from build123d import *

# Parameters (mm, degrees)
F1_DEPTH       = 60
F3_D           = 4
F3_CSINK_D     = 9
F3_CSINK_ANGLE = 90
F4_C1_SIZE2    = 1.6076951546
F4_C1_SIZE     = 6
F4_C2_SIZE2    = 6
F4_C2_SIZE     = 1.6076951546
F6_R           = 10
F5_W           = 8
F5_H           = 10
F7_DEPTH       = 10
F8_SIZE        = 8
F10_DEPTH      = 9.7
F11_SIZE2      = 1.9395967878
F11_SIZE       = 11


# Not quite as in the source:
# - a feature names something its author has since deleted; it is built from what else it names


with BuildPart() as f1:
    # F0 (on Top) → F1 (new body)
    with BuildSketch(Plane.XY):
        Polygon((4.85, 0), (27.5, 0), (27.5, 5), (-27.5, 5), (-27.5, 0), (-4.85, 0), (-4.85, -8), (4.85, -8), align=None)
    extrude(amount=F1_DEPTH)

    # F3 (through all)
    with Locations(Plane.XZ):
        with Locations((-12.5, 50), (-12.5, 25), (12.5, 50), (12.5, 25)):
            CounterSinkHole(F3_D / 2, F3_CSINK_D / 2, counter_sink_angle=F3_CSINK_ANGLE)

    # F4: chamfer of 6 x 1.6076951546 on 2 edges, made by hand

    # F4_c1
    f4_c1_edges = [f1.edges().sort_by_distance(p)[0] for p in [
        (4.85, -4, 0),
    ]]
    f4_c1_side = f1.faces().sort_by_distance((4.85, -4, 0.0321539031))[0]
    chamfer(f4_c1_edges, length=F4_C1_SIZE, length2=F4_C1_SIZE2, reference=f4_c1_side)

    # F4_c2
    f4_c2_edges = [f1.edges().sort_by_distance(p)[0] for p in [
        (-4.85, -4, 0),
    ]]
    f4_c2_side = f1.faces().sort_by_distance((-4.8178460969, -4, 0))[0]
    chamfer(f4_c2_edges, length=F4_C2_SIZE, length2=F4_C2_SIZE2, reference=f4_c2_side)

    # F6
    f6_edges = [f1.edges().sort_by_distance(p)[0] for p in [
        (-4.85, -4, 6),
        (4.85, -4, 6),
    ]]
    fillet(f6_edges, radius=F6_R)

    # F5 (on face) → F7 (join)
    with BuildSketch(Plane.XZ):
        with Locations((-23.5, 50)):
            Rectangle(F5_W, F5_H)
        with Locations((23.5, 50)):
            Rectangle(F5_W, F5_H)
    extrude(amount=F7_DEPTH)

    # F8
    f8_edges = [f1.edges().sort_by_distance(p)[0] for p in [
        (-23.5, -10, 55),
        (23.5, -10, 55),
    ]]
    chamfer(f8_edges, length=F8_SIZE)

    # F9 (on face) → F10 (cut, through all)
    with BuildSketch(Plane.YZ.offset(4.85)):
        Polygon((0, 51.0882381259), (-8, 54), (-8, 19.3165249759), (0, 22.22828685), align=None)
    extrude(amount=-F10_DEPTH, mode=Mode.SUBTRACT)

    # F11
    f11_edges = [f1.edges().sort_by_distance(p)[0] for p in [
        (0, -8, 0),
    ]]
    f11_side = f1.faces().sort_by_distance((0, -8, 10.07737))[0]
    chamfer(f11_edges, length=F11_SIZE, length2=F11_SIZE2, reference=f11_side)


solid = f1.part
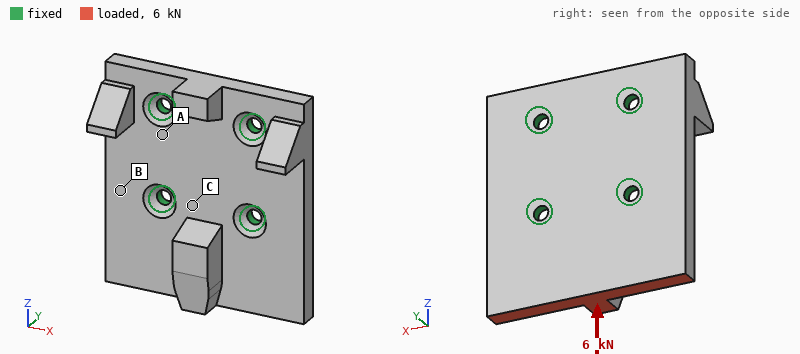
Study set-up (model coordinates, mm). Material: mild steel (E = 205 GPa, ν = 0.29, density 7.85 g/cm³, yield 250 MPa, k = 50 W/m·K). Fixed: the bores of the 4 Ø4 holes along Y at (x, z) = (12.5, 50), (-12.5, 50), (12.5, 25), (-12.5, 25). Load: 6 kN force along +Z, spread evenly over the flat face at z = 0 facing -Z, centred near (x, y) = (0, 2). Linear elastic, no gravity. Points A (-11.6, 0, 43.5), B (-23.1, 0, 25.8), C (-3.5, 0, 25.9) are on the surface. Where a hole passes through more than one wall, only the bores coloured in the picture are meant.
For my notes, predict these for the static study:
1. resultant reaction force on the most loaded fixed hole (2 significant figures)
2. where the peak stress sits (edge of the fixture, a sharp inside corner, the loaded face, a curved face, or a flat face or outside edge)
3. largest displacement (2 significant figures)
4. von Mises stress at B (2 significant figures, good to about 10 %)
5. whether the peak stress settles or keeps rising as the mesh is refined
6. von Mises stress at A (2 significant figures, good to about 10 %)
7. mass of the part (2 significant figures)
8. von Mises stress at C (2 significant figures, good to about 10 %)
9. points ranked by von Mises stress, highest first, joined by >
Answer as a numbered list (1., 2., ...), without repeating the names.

1. 2.1 kN
2. edge of the fixture
3. 19 µm
4. 31 MPa
5. keeps rising
6. 9.1 MPa
7. 150 g
8. 43 MPa
9. C > B > A
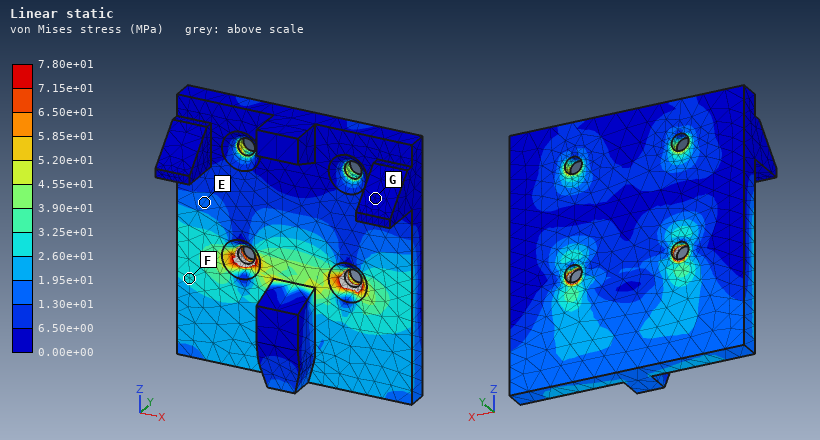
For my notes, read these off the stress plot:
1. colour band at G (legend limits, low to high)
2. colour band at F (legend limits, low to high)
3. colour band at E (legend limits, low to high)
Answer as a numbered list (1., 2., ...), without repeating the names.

1. 0.00e+00 to 6.50e+00 MPa
2. 2.60e+01 to 3.25e+01 MPa
3. 1.30e+01 to 1.95e+01 MPa
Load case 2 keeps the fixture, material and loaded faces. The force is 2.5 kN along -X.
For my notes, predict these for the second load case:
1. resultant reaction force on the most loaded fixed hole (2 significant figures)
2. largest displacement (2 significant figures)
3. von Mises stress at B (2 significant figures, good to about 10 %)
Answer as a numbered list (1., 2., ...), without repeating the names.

1. 2.0 kN
2. 8.3 µm
3. 18 MPa
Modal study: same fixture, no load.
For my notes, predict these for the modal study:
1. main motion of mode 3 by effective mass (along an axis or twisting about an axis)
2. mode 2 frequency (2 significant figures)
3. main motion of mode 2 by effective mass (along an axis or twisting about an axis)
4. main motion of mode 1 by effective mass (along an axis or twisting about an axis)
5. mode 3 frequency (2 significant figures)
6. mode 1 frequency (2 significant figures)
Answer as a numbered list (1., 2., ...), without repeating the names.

1. along Y
2. 7700 Hz
3. twisting about Z
4. along Y
5. 9500 Hz
6. 4600 Hz
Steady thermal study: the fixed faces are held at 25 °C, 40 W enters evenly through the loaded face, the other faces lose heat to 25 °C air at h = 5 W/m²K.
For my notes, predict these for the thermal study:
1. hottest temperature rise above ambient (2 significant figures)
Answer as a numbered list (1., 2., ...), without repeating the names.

1. 78 K
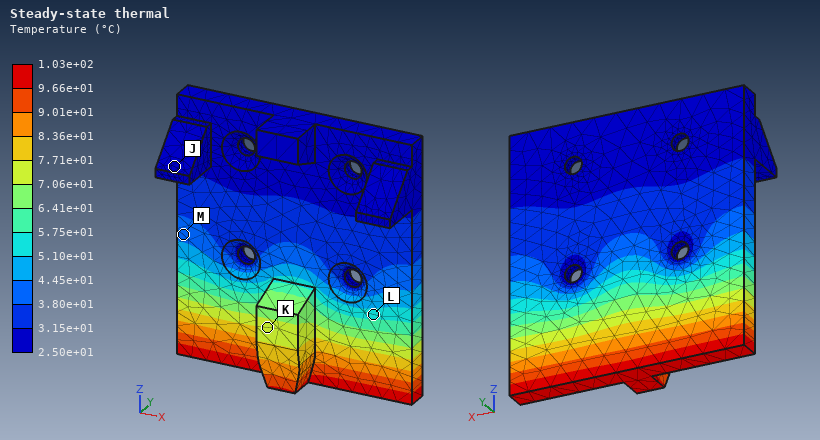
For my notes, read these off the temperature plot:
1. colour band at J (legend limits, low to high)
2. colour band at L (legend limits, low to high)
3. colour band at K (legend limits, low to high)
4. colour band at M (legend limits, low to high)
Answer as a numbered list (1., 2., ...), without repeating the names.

1. 2.50e+01 to 3.15e+01 °C
2. 5.10e+01 to 5.75e+01 °C
3. 7.06e+01 to 7.71e+01 °C
4. 3.80e+01 to 4.45e+01 °C
